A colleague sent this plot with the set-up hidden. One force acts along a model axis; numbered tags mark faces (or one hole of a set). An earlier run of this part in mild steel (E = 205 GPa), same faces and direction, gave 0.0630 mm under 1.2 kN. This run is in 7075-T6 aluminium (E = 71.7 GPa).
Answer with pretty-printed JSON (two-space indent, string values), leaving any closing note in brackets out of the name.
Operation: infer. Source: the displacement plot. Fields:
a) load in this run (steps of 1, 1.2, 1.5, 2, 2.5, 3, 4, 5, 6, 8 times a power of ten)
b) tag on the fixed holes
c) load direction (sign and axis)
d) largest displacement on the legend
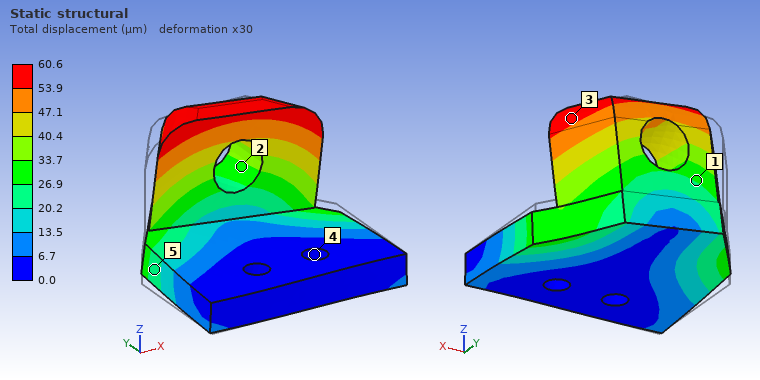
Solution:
{
  "load in this run": "400 N",
  "tag on the fixed holes": "4",
  "load direction": "+X",
  "largest displacement on the legend": "60.6 µm"
}
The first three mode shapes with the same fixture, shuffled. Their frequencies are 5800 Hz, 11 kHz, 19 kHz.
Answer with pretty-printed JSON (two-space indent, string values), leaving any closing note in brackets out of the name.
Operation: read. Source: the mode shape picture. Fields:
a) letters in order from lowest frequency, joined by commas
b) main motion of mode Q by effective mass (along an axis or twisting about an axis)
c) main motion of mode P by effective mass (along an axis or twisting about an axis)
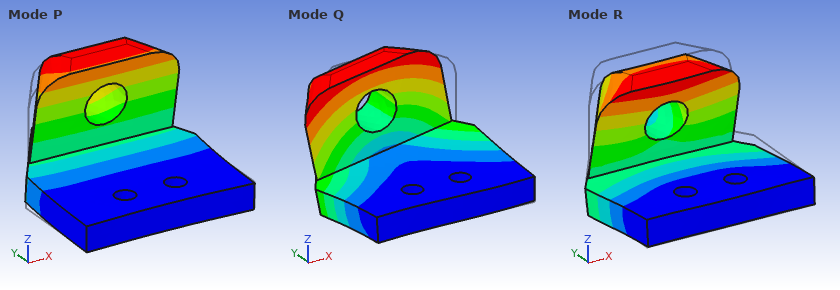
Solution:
{
  "letters in order from lowest frequency, joined by commas": "P, Q, R",
  "main motion of mode Q by effective mass": "along X",
  "main motion of mode P by effective mass": "along Z"
}
